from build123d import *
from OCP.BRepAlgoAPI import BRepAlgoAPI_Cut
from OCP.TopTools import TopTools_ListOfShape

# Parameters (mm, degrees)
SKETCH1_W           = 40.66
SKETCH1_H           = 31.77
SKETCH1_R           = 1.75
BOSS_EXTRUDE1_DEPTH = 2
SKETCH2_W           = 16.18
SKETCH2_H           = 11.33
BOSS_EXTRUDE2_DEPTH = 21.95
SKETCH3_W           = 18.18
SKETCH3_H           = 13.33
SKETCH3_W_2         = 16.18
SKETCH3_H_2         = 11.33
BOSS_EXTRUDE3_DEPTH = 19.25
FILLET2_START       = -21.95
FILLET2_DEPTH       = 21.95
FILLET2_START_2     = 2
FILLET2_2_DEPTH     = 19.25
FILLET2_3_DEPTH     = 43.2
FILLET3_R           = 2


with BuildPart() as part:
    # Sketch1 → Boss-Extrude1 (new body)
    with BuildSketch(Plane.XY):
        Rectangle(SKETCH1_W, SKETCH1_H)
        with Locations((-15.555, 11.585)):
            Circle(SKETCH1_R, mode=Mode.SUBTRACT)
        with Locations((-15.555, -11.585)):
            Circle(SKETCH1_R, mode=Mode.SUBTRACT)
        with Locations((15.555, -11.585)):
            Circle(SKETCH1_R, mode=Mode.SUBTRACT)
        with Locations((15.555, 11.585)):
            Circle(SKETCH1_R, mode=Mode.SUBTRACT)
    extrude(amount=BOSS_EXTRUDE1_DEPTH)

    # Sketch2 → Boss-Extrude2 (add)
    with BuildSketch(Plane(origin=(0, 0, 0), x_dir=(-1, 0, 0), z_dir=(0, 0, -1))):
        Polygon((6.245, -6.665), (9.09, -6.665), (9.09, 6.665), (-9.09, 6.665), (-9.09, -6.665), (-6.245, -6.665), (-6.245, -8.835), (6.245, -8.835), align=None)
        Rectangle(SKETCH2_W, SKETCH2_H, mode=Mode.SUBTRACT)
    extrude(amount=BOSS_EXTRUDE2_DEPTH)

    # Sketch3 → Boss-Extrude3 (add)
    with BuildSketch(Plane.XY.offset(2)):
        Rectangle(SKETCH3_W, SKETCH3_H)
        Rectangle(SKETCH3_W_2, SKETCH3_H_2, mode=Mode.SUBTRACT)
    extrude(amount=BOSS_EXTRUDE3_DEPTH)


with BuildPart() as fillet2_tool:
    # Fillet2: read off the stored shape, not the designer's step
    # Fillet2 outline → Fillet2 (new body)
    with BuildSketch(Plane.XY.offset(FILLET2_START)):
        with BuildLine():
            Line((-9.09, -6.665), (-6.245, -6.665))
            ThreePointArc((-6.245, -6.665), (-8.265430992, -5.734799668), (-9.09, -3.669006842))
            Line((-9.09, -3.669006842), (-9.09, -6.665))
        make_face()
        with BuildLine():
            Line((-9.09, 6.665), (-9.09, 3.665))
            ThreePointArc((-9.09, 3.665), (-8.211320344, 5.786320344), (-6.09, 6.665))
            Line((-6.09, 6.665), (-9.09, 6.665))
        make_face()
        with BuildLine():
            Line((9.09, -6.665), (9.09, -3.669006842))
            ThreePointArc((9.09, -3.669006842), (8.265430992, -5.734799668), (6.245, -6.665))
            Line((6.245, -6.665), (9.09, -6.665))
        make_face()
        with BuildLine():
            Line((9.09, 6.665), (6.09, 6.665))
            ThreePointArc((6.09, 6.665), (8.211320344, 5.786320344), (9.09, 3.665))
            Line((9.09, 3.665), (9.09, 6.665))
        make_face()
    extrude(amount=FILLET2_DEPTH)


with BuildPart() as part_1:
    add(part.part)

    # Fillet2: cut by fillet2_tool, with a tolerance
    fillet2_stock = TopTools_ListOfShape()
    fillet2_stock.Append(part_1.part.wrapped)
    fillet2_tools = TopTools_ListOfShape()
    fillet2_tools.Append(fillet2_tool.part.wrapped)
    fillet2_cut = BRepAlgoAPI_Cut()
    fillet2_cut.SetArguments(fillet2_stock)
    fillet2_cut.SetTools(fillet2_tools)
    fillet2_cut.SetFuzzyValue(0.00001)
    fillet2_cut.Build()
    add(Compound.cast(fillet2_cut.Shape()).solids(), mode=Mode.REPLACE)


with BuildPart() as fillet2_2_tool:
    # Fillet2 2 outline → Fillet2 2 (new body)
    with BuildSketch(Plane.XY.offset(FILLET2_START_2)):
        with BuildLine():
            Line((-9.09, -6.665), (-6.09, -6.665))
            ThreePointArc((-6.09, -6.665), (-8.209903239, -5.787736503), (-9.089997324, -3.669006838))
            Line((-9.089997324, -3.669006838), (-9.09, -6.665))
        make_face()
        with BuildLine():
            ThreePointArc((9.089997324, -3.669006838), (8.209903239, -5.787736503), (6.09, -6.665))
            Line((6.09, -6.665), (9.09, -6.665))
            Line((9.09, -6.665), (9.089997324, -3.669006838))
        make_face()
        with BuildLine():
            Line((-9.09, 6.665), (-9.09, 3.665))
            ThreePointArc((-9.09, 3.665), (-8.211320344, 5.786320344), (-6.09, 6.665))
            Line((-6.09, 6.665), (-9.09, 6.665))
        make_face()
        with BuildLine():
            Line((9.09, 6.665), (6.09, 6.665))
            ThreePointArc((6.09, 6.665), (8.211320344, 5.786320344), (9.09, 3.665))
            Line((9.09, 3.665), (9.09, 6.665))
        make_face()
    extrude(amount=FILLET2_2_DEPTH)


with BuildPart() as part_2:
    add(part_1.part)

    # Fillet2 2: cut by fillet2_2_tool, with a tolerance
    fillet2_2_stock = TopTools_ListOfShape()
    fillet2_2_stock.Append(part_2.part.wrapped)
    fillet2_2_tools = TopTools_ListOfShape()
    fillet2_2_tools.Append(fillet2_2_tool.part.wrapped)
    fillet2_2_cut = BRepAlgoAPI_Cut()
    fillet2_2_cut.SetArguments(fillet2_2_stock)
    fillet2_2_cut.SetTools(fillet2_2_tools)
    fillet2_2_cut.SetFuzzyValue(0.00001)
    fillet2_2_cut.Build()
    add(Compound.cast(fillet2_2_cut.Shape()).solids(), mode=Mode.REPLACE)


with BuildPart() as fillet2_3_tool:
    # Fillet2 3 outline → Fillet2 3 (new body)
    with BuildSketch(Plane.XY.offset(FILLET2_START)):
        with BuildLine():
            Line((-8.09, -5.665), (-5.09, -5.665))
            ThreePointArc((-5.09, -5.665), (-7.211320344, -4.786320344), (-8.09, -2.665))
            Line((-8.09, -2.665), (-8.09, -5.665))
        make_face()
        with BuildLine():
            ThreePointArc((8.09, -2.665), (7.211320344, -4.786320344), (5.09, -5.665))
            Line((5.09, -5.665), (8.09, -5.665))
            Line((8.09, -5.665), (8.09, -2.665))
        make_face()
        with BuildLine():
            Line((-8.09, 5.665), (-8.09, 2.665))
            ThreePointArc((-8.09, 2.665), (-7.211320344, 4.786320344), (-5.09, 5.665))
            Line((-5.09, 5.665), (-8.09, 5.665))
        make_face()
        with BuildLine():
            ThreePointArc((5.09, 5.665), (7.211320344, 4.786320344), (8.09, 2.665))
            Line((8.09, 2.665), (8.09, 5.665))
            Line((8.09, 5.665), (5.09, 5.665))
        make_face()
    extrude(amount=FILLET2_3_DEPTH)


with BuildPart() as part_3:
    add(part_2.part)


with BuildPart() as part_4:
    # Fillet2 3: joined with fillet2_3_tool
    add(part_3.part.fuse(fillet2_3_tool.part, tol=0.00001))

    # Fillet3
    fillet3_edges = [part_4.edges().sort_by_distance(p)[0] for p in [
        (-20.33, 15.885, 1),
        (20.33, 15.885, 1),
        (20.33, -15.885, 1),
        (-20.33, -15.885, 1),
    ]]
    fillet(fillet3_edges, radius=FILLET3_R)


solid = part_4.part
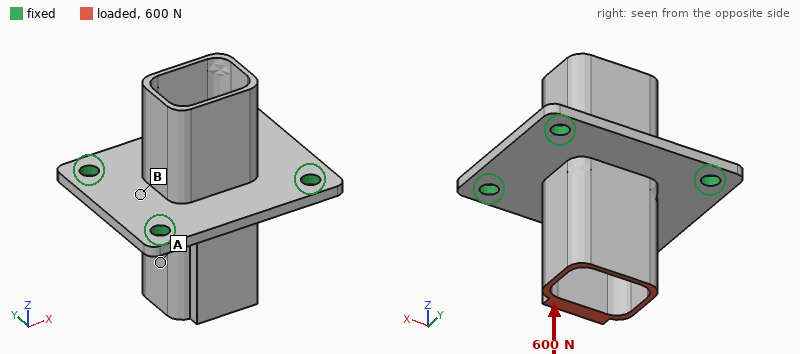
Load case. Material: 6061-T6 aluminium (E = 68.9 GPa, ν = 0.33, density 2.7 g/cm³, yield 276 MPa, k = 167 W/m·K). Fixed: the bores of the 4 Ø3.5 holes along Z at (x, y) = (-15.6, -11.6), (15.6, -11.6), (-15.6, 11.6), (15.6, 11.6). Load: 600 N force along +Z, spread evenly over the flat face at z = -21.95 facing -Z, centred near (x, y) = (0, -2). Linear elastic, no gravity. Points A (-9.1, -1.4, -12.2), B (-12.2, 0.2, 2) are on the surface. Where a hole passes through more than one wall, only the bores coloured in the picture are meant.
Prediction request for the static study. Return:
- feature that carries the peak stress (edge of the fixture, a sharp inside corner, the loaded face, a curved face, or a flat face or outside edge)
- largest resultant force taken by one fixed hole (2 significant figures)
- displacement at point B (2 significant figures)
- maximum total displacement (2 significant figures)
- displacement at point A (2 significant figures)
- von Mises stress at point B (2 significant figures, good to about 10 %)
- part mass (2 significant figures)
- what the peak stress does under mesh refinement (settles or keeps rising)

edge of the fixture
190 N
17 µm
32 µm
25 µm
20 MPa
15 g
keeps rising
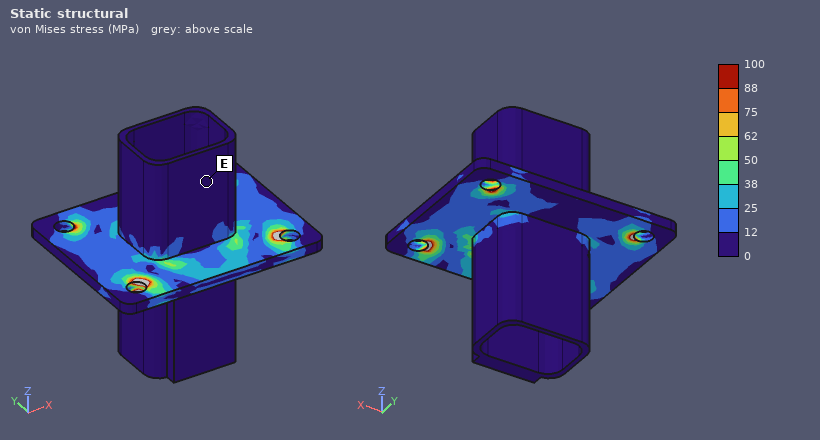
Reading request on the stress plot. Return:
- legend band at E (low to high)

0 to 12 MPa
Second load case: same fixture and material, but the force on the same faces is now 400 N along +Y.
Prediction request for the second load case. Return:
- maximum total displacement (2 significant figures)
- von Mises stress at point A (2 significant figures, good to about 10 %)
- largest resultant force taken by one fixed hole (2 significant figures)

0.15 mm
34 MPa
260 N
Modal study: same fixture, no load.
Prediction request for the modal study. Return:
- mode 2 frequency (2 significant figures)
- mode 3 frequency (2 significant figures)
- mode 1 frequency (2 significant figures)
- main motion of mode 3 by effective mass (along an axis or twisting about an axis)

6900 Hz
7600 Hz
5400 Hz
along Z
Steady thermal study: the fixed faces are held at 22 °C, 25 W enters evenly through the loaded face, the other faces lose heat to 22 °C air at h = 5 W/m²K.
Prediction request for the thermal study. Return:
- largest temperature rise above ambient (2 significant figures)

53 K
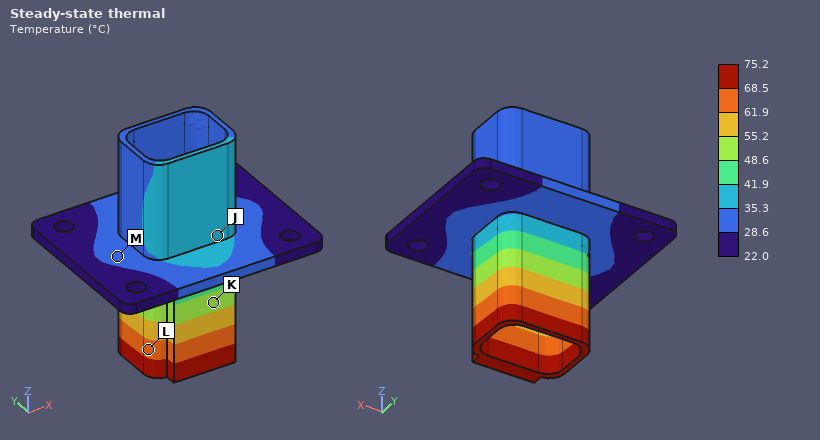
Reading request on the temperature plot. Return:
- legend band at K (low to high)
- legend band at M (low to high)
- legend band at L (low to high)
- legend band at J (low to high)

48.6 to 55.2 °C
28.6 to 35.3 °C
61.9 to 68.5 °C
35.3 to 41.9 °C
